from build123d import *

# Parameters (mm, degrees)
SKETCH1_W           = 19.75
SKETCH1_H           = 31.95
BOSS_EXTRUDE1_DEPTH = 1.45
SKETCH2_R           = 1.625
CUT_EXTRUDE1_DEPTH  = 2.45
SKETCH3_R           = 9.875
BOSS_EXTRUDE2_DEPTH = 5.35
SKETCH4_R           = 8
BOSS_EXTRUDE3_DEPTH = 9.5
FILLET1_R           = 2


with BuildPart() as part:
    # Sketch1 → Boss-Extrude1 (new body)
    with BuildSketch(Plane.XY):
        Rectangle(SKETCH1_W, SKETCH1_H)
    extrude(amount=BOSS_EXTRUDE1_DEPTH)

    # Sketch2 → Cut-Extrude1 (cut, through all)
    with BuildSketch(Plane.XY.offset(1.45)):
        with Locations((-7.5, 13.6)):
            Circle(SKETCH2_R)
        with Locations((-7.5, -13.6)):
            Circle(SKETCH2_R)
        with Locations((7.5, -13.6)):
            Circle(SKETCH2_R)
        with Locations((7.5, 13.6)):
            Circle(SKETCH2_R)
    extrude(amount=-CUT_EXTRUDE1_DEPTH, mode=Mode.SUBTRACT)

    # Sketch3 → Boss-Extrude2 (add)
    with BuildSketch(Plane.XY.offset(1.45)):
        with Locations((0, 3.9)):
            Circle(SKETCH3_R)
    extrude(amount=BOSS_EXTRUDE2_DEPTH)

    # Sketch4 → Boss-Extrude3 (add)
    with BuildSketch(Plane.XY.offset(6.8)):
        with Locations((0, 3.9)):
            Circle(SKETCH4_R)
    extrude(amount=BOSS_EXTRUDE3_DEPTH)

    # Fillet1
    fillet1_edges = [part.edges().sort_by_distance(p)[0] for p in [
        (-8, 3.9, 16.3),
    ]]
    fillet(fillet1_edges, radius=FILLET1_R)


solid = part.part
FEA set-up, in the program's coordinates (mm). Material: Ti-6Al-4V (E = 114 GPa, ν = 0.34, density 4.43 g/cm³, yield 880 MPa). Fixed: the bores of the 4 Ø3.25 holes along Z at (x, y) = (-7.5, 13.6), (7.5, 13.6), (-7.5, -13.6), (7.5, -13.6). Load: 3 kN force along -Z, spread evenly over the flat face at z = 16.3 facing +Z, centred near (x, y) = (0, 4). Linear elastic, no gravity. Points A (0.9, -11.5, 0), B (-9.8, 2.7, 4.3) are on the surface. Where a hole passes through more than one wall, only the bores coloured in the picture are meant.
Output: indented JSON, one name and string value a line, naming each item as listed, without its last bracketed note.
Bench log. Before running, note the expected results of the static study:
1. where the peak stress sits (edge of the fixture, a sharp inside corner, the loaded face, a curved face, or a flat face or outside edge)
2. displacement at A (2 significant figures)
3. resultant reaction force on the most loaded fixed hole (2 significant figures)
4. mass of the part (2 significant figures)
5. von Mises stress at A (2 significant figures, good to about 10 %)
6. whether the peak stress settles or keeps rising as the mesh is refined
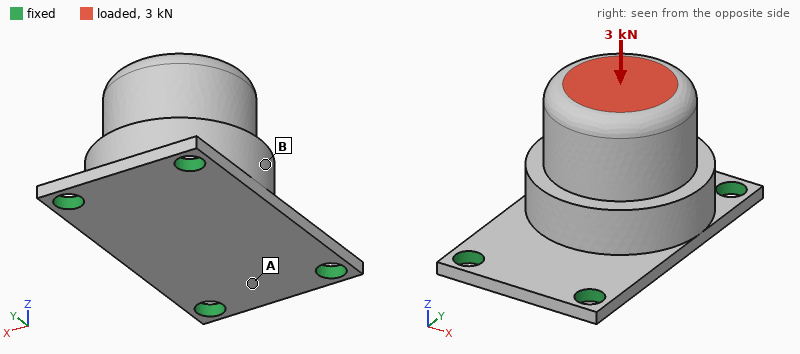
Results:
{
  "where the peak stress sits": "edge of the fixture",
  "displacement at A": "0.039 mm",
  "resultant reaction force on the most loaded fixed hole": "1.1 kN",
  "mass of the part": "19 g",
  "von Mises stress at A": "180 MPa",
  "whether the peak stress settles or keeps rising as the mesh is refined": "keeps rising"
}
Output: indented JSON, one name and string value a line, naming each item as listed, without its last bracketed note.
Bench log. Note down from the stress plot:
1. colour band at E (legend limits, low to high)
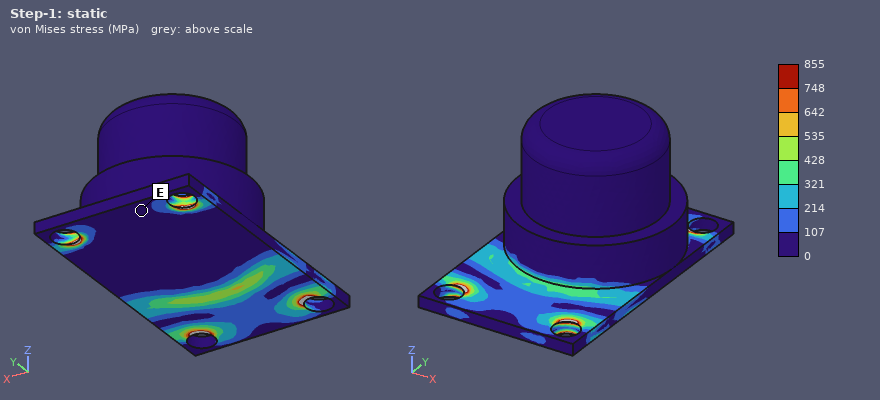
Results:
{
  "colour band at E": "0 to 107 MPa"
}
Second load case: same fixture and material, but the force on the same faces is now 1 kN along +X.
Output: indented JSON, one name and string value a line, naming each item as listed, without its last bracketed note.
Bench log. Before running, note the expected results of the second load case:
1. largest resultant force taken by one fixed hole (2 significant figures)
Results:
{
  "largest resultant force taken by one fixed hole": "1.3 kN"
}
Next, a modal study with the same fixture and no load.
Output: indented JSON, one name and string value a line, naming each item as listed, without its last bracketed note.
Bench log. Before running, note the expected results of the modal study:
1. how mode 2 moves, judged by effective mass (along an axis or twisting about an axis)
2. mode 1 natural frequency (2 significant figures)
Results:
{
  "how mode 2 moves, judged by effective mass": "along X",
  "mode 1 natural frequency": "6100 Hz"
}
